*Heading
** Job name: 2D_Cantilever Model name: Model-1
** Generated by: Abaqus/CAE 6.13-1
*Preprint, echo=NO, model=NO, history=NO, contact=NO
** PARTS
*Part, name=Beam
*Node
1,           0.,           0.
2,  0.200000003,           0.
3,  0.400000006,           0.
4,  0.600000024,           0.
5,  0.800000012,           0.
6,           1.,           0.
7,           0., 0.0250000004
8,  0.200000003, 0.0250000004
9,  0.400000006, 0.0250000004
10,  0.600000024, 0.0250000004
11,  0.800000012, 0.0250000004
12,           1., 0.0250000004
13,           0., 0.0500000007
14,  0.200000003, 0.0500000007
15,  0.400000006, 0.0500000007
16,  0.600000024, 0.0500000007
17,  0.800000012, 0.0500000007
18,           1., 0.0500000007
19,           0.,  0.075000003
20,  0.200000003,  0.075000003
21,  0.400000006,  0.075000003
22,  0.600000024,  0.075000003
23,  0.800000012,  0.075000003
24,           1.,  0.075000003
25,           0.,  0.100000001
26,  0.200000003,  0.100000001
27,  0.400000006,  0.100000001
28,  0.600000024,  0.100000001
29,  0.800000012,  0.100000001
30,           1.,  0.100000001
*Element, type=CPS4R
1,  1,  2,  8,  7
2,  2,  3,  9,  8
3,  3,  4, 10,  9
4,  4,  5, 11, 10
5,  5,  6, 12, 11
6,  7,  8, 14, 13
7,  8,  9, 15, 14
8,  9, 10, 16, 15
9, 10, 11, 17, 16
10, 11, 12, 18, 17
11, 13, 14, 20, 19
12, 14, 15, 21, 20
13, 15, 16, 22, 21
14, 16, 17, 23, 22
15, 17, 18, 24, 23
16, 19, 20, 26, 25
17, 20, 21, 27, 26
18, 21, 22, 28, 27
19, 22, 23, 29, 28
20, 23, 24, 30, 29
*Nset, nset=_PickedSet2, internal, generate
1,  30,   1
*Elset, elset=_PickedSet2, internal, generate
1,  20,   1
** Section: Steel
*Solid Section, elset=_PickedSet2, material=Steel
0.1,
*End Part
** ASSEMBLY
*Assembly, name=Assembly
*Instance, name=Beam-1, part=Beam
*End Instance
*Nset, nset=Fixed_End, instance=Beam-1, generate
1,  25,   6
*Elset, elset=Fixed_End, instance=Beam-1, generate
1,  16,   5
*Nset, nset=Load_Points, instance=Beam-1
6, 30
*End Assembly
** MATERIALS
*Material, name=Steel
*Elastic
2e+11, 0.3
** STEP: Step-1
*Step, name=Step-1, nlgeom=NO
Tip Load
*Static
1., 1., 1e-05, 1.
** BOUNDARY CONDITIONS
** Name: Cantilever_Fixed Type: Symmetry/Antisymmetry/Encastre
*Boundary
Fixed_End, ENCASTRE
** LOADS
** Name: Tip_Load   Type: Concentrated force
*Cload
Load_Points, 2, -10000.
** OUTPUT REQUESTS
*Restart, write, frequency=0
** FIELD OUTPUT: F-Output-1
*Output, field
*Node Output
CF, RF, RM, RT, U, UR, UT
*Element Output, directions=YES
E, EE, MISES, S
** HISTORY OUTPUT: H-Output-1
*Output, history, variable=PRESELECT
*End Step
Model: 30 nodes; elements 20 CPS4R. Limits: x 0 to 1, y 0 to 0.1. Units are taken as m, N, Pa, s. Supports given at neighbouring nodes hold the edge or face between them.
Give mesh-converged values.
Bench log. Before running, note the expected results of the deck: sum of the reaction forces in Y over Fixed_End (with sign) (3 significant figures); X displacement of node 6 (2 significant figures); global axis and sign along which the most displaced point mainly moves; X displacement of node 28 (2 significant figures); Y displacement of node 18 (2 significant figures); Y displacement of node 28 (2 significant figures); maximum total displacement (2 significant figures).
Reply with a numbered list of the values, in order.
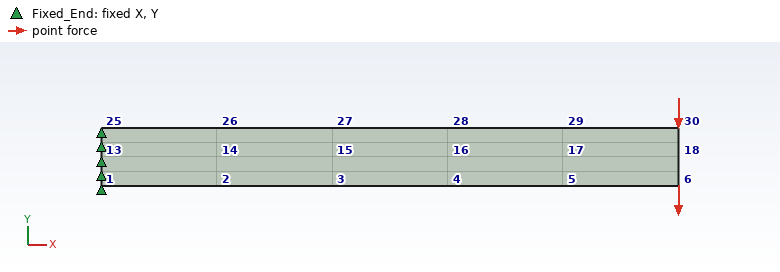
1. 20000 N
2. -2.9e-04 m
3. -Y
4. 2.5e-04 m
5. -0.0039 m
6. -0.0017 m
7. 0.0039 m
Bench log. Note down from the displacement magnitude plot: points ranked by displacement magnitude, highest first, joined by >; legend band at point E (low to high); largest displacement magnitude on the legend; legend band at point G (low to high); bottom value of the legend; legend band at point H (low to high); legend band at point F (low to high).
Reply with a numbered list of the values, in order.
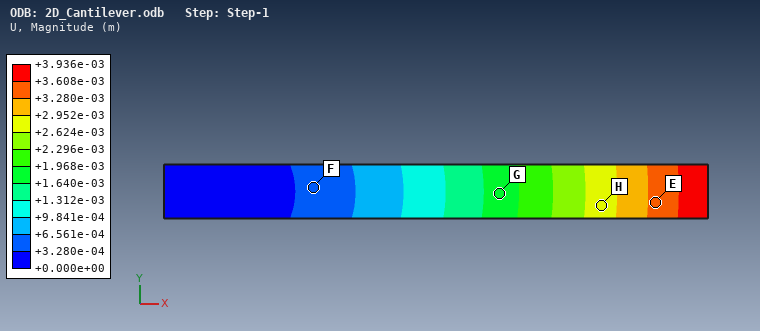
1. E > H > G > F
2. +3.280e-03 to +3.608e-03 m
3. +3.936e-03 m
4. +1.640e-03 to +1.968e-03 m
5. +0.000e+00 m
6. +2.624e-03 to +2.952e-03 m
7. +3.280e-04 to +6.561e-04 m
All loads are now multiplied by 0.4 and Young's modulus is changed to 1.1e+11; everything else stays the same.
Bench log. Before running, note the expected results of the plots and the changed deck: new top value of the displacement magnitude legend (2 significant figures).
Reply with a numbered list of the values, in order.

1. 0.0029 m
